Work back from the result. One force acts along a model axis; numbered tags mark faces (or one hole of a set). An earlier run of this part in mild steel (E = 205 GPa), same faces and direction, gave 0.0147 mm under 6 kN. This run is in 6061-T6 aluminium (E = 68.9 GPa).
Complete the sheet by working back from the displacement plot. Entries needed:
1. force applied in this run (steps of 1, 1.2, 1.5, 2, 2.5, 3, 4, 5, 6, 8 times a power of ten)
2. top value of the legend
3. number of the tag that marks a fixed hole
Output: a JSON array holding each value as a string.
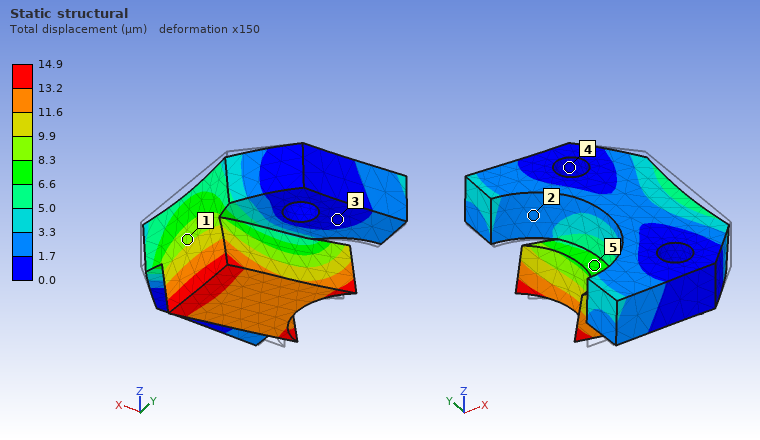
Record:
["2 kN", "14.9 µm", "4"]
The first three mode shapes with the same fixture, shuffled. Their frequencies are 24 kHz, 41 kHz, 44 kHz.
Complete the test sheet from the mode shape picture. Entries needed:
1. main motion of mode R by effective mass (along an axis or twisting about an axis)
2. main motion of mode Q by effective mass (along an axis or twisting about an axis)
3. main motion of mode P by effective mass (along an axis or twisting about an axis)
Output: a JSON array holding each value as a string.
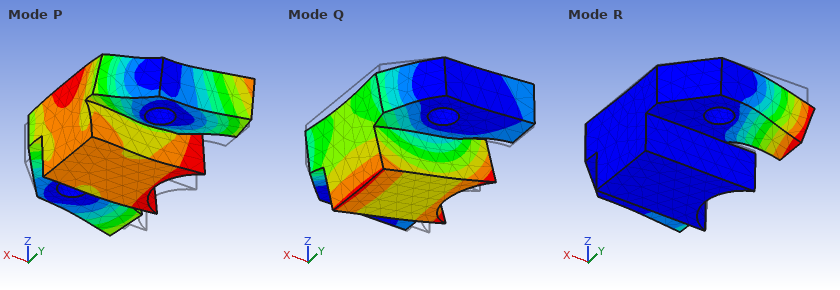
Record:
["along Z", "along X", "along Z"]
